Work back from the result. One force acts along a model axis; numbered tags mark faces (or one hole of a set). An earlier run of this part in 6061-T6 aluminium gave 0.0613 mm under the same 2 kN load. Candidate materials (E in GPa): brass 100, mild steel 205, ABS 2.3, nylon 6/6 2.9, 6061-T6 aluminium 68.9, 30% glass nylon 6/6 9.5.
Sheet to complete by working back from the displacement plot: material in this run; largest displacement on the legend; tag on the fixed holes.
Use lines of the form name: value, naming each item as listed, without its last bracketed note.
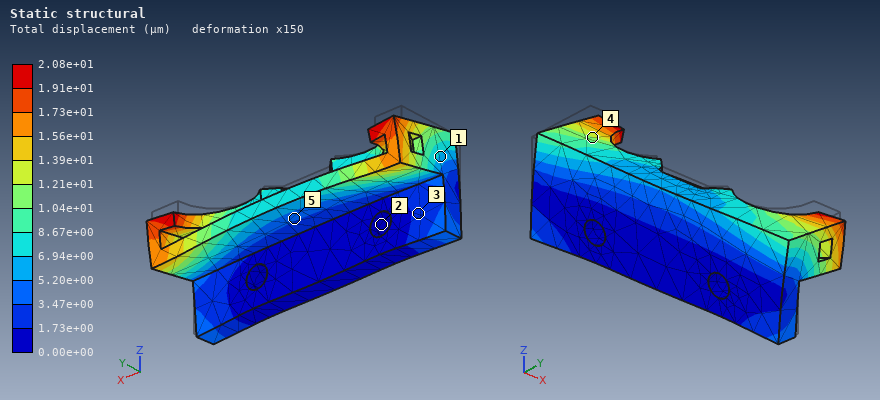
material in this run: mild steel
largest displacement on the legend: 2.08e+01 µm
tag on the fixed holes: 2
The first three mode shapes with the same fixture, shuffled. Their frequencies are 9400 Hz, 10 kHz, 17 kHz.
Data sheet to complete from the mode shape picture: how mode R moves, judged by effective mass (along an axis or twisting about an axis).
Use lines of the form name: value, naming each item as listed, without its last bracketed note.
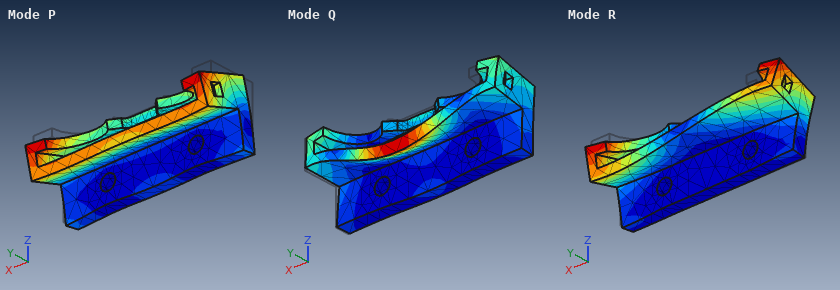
how mode R moves, judged by effective mass: twisting about Z
